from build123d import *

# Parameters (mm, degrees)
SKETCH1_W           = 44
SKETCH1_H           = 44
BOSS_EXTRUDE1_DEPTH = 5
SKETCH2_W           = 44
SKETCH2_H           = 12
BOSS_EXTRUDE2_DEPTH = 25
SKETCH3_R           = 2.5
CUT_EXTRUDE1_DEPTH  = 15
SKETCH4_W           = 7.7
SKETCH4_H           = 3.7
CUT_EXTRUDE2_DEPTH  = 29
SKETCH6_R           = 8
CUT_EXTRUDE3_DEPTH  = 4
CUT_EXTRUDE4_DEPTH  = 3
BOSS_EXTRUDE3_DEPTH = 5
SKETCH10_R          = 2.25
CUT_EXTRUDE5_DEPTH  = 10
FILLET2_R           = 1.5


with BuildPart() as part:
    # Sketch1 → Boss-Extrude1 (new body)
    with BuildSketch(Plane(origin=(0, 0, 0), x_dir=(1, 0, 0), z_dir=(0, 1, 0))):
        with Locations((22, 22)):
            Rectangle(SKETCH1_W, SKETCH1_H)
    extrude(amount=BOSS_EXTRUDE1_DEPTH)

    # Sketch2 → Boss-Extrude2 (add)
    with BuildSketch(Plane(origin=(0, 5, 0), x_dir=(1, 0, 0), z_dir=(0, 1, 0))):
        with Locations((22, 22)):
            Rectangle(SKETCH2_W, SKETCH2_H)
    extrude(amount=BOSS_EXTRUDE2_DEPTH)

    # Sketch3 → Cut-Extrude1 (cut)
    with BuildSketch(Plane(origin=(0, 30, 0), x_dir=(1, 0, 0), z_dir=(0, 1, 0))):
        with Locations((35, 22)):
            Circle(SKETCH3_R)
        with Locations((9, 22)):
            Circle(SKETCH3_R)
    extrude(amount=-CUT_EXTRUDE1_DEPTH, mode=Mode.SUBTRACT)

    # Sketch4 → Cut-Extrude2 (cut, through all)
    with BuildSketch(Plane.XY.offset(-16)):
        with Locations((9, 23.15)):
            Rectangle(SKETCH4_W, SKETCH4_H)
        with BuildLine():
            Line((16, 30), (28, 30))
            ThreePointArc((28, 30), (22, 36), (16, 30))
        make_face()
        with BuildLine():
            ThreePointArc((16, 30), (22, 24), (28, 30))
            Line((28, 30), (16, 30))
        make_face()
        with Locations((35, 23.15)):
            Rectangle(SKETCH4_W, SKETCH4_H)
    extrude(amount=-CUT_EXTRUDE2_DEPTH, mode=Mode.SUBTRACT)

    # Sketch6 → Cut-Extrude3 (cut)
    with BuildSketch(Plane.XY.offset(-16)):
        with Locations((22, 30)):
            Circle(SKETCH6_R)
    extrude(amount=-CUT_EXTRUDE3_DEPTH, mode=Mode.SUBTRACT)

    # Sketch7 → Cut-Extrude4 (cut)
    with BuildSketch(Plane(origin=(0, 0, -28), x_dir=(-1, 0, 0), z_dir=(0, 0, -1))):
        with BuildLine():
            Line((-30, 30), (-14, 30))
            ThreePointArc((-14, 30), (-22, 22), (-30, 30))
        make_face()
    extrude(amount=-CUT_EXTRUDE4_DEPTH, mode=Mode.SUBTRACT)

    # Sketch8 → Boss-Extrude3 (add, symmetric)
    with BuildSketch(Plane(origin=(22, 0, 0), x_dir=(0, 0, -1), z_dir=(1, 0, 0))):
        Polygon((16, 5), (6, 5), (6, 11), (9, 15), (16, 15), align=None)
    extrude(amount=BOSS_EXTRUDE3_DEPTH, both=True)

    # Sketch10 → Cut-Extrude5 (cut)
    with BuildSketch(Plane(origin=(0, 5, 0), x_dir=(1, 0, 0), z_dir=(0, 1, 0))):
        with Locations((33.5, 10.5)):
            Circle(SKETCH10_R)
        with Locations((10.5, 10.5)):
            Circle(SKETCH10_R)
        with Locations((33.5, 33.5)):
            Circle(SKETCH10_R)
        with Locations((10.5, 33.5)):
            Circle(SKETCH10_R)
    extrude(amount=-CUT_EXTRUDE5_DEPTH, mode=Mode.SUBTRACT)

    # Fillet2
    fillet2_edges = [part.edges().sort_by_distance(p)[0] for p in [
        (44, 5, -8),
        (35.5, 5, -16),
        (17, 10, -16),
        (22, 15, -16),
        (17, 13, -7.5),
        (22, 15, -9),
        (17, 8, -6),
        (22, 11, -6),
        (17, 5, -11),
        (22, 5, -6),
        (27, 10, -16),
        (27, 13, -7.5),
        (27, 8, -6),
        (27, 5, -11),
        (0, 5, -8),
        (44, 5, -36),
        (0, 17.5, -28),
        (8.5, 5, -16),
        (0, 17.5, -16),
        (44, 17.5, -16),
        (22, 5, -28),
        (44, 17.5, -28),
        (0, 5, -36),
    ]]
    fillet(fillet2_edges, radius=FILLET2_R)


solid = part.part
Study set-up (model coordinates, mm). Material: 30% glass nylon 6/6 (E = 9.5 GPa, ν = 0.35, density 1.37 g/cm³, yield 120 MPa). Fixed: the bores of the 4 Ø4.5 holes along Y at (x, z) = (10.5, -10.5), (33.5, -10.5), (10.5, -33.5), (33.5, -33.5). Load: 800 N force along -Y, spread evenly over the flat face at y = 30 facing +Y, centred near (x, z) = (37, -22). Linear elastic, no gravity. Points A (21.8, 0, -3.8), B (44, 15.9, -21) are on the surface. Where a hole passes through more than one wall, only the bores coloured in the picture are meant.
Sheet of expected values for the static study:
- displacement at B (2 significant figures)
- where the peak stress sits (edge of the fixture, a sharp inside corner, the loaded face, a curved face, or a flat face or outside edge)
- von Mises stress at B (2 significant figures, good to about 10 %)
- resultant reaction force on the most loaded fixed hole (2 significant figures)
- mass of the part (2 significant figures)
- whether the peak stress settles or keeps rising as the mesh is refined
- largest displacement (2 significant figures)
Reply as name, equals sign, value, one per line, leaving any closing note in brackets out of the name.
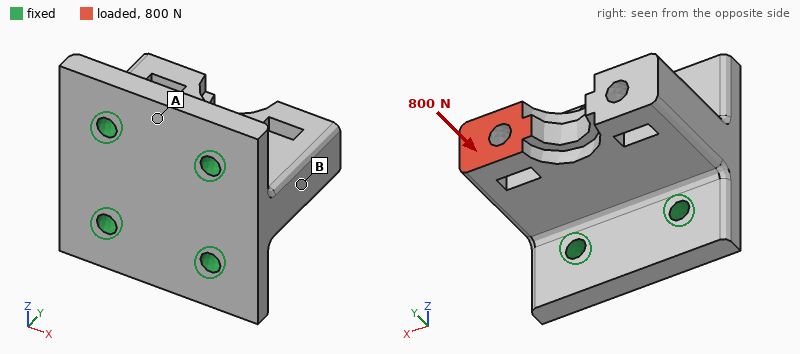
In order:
displacement at B = 37 µm
where the peak stress sits = edge of the fixture
von Mises stress at B = 7.7 MPa
resultant reaction force on the most loaded fixed hole = 460 N
mass of the part = 29 g
whether the peak stress settles or keeps rising as the mesh is refined = keeps rising
largest displacement = 52 µm
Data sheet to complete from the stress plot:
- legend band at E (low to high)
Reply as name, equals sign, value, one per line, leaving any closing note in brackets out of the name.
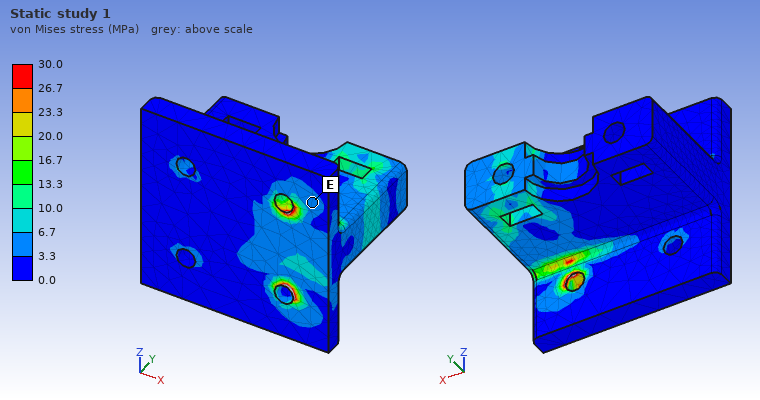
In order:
legend band at E = 3.3 to 6.7 MPa
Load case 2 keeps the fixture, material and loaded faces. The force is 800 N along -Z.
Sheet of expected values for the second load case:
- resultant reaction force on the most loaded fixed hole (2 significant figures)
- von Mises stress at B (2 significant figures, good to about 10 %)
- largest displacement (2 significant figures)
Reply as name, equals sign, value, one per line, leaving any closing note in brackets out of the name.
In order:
resultant reaction force on the most loaded fixed hole = 770 N
von Mises stress at B = 9.5 MPa
largest displacement = 0.26 mm
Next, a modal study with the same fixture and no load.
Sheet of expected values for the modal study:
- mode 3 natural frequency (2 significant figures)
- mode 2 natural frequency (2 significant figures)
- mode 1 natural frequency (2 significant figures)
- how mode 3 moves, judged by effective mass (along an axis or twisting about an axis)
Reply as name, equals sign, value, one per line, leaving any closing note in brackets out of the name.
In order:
mode 3 natural frequency = 8500 Hz
mode 2 natural frequency = 6600 Hz
mode 1 natural frequency = 6500 Hz
how mode 3 moves, judged by effective mass = twisting about Y
